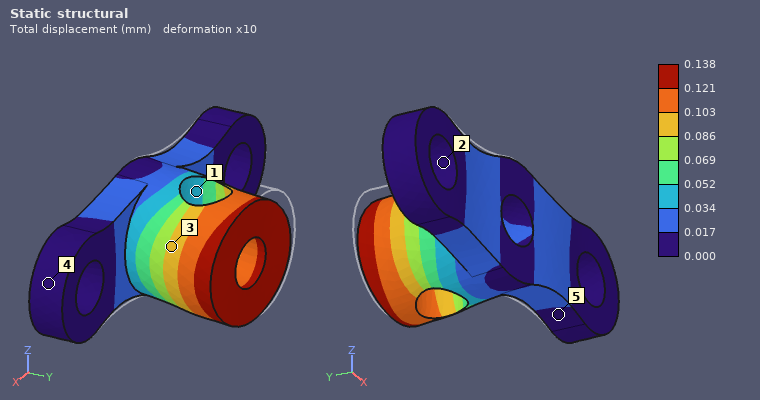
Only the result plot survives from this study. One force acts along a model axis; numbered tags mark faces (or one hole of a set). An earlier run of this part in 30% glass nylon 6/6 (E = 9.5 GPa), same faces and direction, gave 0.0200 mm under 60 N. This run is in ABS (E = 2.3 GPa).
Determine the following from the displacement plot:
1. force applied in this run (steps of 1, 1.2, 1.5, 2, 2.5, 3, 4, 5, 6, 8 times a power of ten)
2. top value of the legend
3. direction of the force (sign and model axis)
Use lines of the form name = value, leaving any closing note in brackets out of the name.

force applied in this run = 100 N
top value of the legend = 0.138 mm
direction of the force = +X
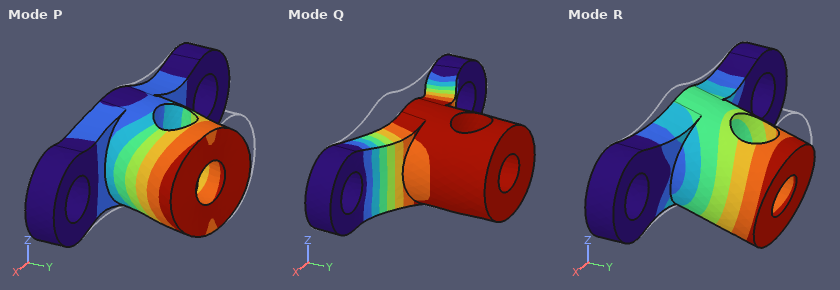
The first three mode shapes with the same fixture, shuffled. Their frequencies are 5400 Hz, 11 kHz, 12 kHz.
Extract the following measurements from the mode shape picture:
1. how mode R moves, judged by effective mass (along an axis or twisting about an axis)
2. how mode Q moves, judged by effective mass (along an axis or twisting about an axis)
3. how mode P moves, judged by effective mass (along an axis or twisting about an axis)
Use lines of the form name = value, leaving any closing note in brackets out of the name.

how mode R moves, judged by effective mass = along Z
how mode Q moves, judged by effective mass = along Y
how mode P moves, judged by effective mass = along X
